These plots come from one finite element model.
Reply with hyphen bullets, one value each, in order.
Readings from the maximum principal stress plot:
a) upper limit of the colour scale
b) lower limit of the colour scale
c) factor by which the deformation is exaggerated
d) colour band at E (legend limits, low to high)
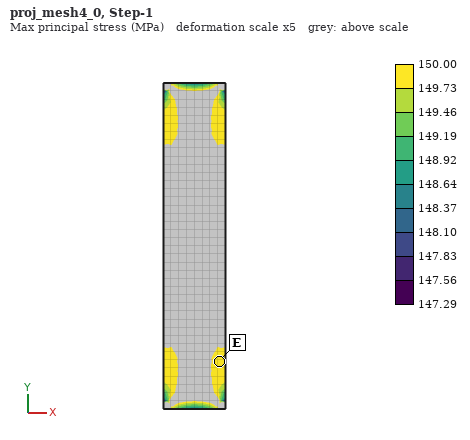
- 150.00 MPa
- 147.29 MPa
- 5
- 149.73 to 150.00 MPa
